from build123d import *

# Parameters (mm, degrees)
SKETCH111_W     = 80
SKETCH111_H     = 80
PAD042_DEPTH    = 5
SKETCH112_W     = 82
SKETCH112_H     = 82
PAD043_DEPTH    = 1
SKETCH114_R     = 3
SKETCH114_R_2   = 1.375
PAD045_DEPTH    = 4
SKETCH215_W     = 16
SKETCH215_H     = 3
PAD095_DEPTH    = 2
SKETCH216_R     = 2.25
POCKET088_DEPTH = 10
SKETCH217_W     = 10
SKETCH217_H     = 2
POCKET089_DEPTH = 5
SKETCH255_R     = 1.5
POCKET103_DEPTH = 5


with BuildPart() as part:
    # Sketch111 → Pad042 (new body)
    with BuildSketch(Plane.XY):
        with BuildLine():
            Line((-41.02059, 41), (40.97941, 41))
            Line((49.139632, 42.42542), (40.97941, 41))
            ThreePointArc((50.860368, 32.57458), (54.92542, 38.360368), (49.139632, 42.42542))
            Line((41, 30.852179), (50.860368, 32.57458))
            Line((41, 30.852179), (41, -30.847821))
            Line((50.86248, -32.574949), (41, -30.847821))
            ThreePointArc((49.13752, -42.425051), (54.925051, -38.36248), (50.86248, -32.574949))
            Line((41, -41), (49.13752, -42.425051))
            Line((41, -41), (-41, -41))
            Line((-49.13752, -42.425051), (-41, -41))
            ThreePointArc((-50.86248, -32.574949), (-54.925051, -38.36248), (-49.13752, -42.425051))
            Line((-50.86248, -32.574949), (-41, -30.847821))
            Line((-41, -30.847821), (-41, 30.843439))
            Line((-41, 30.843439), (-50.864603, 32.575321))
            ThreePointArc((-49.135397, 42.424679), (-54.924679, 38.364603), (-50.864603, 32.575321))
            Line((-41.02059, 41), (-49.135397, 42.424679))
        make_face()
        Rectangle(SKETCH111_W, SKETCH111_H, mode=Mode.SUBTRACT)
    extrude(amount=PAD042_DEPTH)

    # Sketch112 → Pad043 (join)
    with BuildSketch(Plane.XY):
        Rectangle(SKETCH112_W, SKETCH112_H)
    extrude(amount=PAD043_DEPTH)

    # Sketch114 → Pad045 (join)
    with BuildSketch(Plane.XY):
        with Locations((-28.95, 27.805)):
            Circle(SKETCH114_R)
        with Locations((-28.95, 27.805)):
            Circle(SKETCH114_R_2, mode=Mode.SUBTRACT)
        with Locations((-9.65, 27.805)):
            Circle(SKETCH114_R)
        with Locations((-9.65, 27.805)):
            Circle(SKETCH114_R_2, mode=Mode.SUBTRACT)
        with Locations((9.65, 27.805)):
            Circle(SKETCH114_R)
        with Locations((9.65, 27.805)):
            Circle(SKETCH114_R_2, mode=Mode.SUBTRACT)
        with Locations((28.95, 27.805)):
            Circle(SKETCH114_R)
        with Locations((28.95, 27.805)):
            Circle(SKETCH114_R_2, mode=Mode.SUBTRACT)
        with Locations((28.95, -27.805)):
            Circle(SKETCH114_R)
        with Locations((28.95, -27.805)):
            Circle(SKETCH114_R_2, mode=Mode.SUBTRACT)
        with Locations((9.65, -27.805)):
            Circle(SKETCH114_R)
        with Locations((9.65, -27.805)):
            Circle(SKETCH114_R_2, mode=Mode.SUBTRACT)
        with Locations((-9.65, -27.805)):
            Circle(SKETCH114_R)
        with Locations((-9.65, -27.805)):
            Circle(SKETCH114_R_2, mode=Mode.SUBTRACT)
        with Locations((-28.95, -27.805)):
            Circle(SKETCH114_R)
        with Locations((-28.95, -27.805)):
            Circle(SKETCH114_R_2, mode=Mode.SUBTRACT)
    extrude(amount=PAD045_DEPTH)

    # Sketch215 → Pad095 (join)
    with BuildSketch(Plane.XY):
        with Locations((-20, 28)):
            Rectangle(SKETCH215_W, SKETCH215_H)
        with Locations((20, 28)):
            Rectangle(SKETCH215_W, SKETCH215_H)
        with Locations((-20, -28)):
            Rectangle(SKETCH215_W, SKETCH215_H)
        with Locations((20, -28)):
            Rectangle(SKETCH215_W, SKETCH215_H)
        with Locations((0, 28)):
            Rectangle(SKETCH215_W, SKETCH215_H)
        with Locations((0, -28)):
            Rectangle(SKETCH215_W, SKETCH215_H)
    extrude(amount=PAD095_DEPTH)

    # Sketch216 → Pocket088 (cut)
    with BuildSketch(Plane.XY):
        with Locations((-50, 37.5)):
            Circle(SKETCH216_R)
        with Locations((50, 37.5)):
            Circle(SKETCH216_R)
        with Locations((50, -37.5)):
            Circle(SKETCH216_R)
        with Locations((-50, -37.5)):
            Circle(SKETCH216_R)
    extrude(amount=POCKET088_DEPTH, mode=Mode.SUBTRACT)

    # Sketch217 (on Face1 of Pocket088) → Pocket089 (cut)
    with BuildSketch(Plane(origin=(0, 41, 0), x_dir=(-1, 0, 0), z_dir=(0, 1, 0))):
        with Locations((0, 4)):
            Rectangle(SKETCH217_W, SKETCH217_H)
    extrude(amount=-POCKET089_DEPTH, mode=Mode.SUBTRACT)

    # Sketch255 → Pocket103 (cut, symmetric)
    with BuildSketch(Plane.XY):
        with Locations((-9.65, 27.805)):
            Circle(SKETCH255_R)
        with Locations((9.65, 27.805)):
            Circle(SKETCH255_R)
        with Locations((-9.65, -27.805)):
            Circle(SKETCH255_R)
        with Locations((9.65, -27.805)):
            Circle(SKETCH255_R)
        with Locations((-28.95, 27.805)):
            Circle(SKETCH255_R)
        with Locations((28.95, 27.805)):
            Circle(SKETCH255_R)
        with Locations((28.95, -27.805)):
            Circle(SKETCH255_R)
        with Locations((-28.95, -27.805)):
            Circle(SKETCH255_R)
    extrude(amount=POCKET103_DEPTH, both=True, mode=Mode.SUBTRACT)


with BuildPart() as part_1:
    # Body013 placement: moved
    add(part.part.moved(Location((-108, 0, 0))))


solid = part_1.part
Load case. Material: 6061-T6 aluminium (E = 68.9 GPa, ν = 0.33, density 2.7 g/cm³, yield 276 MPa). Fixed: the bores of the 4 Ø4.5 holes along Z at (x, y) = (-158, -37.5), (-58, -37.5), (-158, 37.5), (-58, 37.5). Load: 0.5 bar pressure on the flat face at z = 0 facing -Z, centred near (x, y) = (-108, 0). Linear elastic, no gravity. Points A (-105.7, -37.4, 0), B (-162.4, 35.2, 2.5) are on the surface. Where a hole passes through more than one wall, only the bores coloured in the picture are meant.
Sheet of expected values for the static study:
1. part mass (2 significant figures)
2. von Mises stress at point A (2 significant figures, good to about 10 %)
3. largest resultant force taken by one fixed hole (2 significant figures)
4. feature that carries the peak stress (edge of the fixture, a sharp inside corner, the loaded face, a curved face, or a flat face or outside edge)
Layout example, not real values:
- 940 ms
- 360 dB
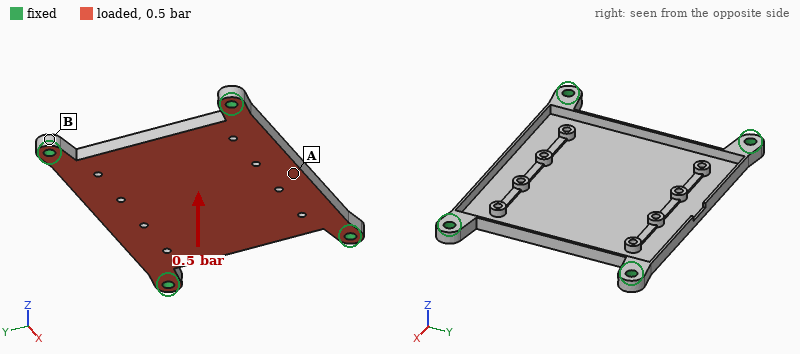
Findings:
- 30 g
- 27 MPa
- 180 N
- a flat face or outside edge
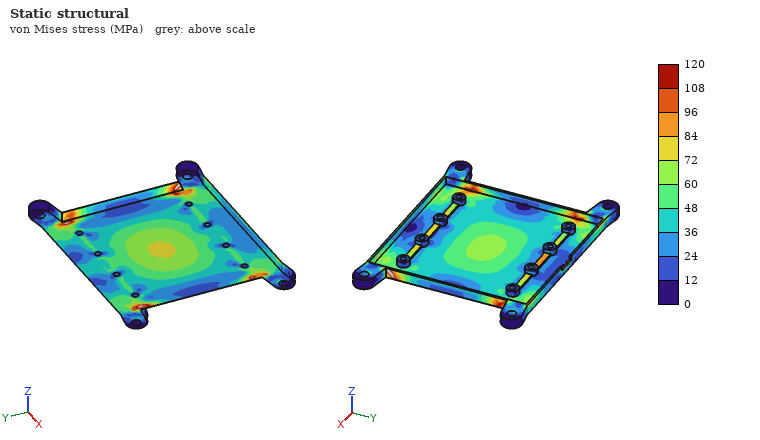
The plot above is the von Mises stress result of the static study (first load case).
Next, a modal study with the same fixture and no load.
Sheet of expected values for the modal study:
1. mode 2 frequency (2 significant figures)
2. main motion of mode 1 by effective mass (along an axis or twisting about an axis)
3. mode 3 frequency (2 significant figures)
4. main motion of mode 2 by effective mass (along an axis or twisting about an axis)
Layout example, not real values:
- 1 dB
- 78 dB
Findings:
- 1700 Hz
- along Z
- 2100 Hz
- twisting about X
